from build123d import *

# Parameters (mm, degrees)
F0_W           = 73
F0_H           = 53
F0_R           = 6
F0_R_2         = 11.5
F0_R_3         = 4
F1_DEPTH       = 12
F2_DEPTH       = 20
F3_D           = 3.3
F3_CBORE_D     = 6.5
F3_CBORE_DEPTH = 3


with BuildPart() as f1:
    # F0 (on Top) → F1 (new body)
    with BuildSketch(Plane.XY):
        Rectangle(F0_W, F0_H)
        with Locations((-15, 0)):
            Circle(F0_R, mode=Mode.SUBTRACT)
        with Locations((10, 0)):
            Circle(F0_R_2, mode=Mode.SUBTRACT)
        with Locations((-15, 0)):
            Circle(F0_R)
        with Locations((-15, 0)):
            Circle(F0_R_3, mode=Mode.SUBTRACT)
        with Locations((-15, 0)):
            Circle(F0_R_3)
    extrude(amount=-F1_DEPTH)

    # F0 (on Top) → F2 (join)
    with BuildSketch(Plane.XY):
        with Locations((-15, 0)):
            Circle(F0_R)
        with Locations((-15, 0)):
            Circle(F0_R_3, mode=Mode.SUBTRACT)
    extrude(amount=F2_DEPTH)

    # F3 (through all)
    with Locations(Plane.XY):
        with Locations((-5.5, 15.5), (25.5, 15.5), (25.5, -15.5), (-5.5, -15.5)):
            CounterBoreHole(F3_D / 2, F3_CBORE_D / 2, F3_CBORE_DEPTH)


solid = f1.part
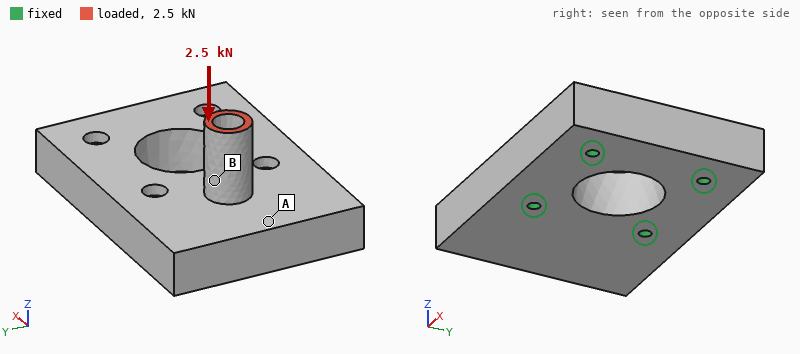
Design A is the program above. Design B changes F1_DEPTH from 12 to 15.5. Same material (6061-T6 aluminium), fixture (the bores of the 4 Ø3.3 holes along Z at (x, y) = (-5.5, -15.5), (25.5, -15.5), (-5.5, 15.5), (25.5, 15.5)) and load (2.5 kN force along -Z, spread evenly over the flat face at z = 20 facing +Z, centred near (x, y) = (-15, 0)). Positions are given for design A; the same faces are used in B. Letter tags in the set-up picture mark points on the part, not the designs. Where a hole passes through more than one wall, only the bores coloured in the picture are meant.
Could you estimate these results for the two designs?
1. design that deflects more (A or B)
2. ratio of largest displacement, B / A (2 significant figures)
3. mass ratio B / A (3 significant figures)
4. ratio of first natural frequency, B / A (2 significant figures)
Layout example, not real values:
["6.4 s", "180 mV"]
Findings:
["A", "0.68", "1.28", "1.2"]
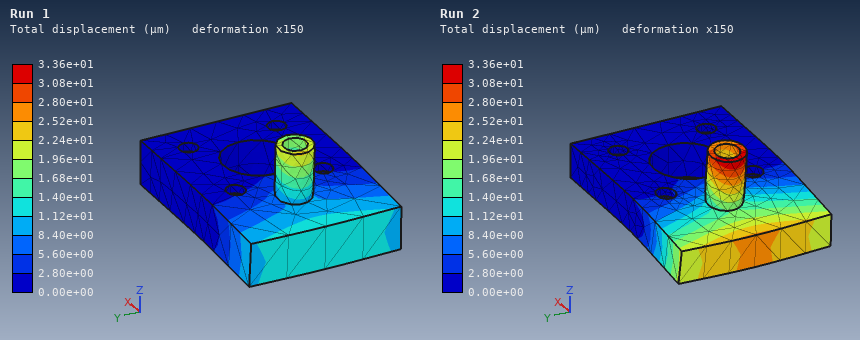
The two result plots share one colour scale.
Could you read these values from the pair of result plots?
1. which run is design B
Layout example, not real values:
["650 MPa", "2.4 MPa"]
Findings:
["Run 1"]
